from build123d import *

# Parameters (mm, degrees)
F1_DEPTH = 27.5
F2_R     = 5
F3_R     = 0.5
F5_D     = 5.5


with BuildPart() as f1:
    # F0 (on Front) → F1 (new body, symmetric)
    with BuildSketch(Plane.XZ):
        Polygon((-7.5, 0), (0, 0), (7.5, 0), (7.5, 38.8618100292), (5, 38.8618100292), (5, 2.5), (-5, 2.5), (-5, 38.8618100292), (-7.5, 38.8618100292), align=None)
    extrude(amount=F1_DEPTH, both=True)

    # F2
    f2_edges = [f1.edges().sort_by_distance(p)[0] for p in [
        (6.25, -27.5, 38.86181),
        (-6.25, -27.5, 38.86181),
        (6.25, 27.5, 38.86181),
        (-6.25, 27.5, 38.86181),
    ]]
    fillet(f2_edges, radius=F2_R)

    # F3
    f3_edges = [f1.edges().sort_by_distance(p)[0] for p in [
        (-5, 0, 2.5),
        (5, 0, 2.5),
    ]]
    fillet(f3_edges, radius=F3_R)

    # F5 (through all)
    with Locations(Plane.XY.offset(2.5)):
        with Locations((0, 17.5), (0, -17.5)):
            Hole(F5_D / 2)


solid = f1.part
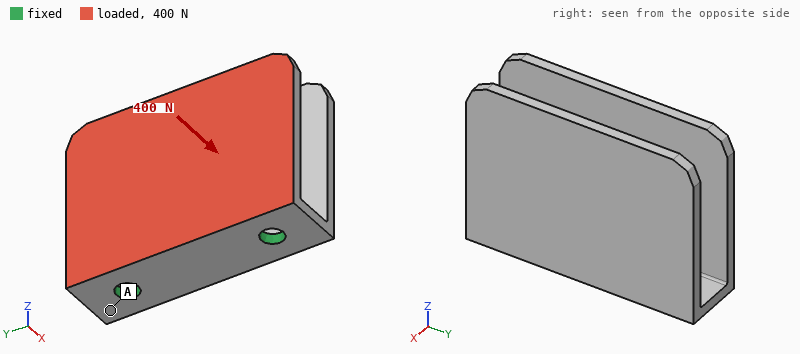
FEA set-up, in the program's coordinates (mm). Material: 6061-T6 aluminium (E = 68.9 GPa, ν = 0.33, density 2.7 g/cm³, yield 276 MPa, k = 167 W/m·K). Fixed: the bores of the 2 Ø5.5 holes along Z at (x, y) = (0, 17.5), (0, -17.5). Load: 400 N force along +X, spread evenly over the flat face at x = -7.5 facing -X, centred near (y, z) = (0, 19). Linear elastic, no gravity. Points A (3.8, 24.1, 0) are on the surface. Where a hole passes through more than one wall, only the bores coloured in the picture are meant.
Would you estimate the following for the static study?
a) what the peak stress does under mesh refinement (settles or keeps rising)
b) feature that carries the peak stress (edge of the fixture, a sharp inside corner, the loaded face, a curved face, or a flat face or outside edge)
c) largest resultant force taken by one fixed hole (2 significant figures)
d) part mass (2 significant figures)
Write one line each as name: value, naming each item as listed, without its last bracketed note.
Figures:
what the peak stress does under mesh refinement: keeps rising
feature that carries the peak stress: edge of the fixture
largest resultant force taken by one fixed hole: 200 N
part mass: 32 g
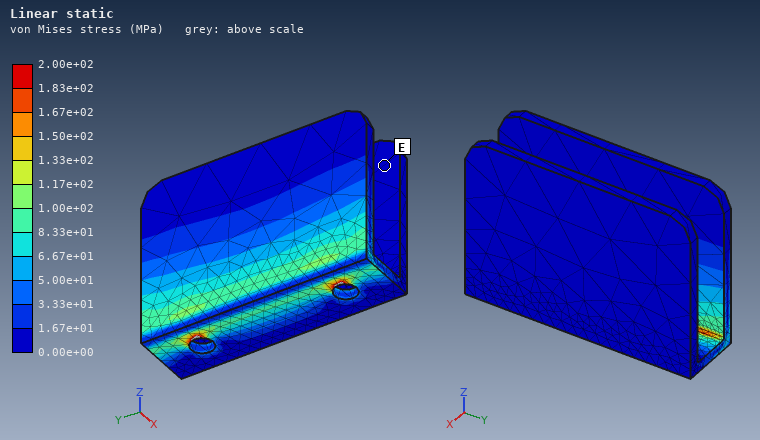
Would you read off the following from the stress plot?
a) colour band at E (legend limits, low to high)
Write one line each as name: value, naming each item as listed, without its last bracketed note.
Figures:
colour band at E: 0.00e+00 to 1.67e+01 MPa
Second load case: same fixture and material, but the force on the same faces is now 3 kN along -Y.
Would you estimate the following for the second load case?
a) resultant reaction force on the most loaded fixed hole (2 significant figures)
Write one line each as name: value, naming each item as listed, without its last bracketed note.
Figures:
resultant reaction force on the most loaded fixed hole: 2.2 kN
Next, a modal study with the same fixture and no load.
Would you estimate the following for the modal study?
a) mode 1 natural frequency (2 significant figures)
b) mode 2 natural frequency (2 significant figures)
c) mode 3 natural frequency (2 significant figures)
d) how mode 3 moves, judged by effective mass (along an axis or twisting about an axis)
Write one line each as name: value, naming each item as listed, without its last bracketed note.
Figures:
mode 1 natural frequency: 1200 Hz
mode 2 natural frequency: 1300 Hz
mode 3 natural frequency: 2500 Hz
how mode 3 moves, judged by effective mass: twisting about Z
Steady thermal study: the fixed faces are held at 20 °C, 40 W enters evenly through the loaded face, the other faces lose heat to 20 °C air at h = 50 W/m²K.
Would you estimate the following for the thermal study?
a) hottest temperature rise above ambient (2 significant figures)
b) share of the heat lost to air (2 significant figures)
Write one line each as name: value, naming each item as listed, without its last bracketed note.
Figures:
hottest temperature rise above ambient: 39 K
share of the heat lost to air: 12 %
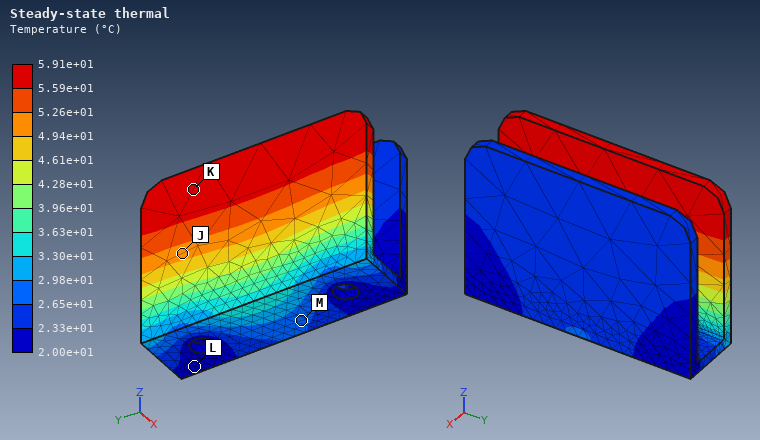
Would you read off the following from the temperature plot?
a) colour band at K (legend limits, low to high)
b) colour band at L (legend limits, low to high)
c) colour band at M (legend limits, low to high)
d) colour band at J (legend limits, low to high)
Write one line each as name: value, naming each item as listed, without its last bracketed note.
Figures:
colour band at K: 5.59e+01 to 5.91e+01 °C
colour band at L: 2.00e+01 to 2.33e+01 °C
colour band at M: 2.65e+01 to 2.98e+01 °C
colour band at J: 4.94e+01 to 5.26e+01 °C
